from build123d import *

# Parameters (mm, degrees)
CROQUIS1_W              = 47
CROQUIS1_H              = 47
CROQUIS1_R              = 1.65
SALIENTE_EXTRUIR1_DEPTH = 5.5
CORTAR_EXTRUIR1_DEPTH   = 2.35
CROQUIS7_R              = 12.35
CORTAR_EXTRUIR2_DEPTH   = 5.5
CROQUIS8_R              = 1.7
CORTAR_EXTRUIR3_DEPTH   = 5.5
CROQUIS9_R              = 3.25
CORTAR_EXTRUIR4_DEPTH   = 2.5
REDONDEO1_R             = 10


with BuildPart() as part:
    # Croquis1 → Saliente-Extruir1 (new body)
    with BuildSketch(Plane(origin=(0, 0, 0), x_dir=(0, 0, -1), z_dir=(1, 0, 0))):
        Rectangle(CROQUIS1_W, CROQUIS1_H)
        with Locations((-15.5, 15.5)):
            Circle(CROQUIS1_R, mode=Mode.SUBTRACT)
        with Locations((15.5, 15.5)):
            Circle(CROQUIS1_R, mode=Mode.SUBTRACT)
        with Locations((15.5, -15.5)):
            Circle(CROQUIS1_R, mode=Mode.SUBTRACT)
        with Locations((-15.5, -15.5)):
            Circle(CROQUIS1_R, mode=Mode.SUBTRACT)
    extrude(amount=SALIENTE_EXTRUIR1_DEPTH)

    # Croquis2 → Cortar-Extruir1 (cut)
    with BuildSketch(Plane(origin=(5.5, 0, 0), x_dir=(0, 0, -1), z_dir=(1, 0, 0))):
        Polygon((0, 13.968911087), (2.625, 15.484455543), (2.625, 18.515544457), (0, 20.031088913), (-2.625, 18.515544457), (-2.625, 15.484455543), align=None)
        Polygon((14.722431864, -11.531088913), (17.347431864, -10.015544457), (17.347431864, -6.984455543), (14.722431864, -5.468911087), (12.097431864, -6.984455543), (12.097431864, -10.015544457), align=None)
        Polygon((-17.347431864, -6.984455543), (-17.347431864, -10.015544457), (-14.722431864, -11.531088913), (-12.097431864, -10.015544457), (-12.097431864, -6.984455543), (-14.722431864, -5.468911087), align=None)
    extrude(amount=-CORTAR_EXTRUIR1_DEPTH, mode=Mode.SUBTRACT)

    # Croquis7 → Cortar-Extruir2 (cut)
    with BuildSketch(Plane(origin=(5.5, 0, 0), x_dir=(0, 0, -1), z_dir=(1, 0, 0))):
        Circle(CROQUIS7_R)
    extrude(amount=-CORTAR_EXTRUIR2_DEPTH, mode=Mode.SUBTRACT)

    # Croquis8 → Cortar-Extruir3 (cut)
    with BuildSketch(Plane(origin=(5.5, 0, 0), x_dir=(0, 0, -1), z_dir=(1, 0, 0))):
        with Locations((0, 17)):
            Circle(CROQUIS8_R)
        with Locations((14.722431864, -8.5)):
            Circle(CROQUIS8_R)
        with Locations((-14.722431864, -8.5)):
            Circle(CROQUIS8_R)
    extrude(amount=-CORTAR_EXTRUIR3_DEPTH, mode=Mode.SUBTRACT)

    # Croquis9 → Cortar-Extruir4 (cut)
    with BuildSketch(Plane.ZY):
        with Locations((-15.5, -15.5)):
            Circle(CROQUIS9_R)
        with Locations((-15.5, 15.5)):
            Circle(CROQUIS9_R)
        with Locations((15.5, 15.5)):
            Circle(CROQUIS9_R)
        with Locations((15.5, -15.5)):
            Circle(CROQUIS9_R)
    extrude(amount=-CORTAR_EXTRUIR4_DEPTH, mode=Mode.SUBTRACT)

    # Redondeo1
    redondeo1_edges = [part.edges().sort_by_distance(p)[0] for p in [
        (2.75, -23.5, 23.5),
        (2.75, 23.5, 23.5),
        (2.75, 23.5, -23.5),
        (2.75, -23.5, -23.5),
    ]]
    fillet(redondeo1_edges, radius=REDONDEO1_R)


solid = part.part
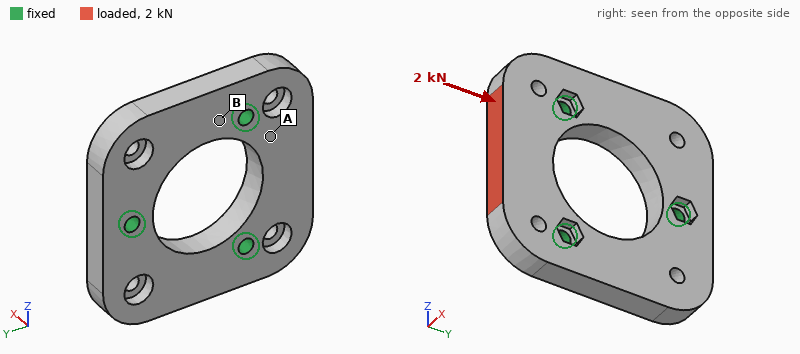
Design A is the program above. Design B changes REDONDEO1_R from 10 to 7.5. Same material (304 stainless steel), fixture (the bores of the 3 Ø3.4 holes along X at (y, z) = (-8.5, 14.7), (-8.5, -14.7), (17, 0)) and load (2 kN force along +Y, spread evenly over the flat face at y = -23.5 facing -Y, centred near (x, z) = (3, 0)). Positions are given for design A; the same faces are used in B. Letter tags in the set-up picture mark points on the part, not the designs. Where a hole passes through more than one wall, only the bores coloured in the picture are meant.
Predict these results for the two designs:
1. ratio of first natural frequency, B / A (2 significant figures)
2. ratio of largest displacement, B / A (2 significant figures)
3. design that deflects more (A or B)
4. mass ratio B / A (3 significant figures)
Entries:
0.96
0.92
A
1.02
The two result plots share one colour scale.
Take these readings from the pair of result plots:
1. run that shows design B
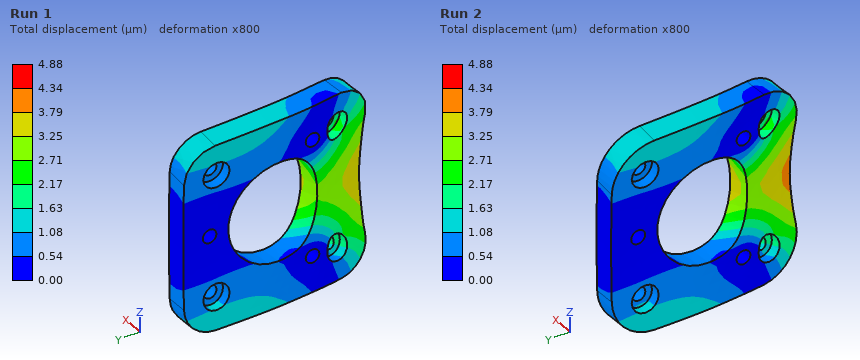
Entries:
Run 1
